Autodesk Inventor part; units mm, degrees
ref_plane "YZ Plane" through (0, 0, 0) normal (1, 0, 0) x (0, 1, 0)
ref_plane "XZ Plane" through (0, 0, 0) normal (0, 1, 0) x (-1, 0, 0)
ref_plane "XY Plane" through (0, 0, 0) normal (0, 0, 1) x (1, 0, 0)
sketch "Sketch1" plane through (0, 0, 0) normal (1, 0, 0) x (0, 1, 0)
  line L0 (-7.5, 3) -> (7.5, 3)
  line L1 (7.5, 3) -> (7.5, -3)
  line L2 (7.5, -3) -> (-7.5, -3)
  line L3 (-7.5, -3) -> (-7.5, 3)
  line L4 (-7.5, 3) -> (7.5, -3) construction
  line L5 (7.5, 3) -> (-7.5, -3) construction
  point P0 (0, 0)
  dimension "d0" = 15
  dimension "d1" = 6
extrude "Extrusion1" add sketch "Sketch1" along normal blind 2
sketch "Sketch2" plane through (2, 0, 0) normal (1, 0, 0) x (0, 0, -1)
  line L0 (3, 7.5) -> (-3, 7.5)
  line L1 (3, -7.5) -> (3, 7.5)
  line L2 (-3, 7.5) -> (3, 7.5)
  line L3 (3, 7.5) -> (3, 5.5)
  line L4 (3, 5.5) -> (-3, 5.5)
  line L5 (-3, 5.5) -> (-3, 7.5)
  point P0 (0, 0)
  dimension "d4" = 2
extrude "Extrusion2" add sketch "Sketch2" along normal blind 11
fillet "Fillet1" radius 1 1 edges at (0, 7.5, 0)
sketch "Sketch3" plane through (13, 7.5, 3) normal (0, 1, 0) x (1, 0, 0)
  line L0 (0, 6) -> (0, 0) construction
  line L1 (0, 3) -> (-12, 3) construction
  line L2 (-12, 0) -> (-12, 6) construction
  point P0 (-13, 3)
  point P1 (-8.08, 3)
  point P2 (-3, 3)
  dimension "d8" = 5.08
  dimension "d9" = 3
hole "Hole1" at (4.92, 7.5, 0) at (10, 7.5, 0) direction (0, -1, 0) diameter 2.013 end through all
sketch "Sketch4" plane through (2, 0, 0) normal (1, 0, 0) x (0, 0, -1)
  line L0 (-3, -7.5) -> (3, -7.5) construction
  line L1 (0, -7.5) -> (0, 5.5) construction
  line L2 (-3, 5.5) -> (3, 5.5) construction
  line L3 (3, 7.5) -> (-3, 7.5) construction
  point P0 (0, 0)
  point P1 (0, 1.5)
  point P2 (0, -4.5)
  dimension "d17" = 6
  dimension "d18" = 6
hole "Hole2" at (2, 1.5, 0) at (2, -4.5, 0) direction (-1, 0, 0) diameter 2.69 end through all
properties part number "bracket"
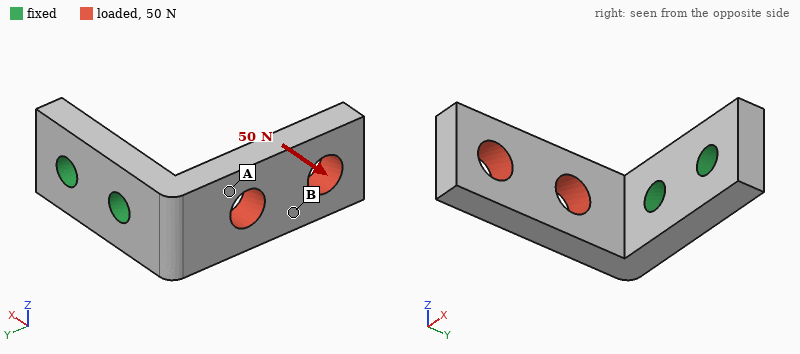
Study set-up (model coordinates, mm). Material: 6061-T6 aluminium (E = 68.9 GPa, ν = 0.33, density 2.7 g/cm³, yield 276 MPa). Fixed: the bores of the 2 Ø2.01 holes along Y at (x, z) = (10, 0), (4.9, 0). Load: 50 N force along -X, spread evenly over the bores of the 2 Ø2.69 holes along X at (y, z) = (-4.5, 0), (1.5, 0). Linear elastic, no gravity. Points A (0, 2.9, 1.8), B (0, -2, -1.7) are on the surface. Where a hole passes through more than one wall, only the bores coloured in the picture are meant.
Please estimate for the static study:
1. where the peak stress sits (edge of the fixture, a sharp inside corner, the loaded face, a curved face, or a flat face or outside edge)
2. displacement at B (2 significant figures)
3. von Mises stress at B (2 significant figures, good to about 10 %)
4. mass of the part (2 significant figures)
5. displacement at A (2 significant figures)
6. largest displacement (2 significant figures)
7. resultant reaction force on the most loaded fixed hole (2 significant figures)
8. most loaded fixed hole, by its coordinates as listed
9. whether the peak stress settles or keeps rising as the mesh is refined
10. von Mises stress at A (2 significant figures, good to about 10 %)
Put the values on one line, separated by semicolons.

edge of the fixture; 0.078 mm; 19 MPa; 0.74 g; 0.028 mm; 0.14 mm; 47 N; (4.9, 0); keeps rising; 80 MPa
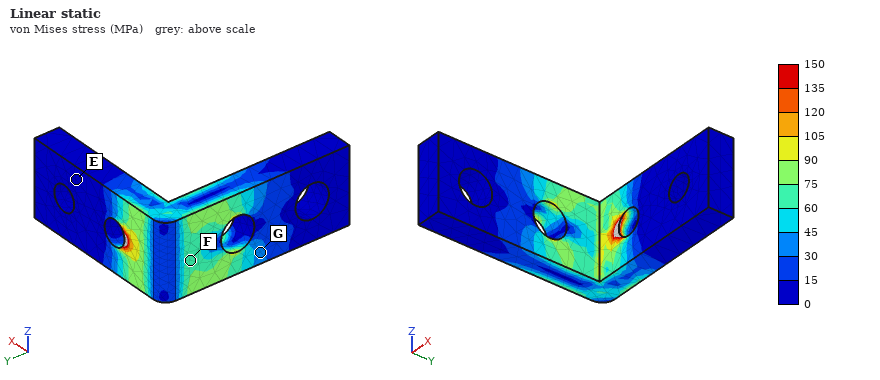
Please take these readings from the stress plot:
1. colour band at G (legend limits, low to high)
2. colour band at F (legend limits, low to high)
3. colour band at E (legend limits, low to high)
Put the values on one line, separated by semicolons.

30 to 45 MPa; 60 to 75 MPa; 0 to 15 MPa
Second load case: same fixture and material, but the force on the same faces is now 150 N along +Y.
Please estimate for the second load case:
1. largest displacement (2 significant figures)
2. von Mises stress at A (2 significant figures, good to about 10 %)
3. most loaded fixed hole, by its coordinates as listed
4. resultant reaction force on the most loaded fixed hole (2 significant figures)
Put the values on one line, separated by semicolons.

51 µm; 19 MPa; (4.9, 0); 170 N
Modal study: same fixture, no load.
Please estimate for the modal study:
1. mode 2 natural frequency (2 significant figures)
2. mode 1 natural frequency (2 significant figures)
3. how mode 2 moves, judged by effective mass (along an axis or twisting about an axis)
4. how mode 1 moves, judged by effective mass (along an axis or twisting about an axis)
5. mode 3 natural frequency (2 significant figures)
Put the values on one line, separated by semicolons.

10 kHz; 6300 Hz; along Z; along X; 28 kHz
